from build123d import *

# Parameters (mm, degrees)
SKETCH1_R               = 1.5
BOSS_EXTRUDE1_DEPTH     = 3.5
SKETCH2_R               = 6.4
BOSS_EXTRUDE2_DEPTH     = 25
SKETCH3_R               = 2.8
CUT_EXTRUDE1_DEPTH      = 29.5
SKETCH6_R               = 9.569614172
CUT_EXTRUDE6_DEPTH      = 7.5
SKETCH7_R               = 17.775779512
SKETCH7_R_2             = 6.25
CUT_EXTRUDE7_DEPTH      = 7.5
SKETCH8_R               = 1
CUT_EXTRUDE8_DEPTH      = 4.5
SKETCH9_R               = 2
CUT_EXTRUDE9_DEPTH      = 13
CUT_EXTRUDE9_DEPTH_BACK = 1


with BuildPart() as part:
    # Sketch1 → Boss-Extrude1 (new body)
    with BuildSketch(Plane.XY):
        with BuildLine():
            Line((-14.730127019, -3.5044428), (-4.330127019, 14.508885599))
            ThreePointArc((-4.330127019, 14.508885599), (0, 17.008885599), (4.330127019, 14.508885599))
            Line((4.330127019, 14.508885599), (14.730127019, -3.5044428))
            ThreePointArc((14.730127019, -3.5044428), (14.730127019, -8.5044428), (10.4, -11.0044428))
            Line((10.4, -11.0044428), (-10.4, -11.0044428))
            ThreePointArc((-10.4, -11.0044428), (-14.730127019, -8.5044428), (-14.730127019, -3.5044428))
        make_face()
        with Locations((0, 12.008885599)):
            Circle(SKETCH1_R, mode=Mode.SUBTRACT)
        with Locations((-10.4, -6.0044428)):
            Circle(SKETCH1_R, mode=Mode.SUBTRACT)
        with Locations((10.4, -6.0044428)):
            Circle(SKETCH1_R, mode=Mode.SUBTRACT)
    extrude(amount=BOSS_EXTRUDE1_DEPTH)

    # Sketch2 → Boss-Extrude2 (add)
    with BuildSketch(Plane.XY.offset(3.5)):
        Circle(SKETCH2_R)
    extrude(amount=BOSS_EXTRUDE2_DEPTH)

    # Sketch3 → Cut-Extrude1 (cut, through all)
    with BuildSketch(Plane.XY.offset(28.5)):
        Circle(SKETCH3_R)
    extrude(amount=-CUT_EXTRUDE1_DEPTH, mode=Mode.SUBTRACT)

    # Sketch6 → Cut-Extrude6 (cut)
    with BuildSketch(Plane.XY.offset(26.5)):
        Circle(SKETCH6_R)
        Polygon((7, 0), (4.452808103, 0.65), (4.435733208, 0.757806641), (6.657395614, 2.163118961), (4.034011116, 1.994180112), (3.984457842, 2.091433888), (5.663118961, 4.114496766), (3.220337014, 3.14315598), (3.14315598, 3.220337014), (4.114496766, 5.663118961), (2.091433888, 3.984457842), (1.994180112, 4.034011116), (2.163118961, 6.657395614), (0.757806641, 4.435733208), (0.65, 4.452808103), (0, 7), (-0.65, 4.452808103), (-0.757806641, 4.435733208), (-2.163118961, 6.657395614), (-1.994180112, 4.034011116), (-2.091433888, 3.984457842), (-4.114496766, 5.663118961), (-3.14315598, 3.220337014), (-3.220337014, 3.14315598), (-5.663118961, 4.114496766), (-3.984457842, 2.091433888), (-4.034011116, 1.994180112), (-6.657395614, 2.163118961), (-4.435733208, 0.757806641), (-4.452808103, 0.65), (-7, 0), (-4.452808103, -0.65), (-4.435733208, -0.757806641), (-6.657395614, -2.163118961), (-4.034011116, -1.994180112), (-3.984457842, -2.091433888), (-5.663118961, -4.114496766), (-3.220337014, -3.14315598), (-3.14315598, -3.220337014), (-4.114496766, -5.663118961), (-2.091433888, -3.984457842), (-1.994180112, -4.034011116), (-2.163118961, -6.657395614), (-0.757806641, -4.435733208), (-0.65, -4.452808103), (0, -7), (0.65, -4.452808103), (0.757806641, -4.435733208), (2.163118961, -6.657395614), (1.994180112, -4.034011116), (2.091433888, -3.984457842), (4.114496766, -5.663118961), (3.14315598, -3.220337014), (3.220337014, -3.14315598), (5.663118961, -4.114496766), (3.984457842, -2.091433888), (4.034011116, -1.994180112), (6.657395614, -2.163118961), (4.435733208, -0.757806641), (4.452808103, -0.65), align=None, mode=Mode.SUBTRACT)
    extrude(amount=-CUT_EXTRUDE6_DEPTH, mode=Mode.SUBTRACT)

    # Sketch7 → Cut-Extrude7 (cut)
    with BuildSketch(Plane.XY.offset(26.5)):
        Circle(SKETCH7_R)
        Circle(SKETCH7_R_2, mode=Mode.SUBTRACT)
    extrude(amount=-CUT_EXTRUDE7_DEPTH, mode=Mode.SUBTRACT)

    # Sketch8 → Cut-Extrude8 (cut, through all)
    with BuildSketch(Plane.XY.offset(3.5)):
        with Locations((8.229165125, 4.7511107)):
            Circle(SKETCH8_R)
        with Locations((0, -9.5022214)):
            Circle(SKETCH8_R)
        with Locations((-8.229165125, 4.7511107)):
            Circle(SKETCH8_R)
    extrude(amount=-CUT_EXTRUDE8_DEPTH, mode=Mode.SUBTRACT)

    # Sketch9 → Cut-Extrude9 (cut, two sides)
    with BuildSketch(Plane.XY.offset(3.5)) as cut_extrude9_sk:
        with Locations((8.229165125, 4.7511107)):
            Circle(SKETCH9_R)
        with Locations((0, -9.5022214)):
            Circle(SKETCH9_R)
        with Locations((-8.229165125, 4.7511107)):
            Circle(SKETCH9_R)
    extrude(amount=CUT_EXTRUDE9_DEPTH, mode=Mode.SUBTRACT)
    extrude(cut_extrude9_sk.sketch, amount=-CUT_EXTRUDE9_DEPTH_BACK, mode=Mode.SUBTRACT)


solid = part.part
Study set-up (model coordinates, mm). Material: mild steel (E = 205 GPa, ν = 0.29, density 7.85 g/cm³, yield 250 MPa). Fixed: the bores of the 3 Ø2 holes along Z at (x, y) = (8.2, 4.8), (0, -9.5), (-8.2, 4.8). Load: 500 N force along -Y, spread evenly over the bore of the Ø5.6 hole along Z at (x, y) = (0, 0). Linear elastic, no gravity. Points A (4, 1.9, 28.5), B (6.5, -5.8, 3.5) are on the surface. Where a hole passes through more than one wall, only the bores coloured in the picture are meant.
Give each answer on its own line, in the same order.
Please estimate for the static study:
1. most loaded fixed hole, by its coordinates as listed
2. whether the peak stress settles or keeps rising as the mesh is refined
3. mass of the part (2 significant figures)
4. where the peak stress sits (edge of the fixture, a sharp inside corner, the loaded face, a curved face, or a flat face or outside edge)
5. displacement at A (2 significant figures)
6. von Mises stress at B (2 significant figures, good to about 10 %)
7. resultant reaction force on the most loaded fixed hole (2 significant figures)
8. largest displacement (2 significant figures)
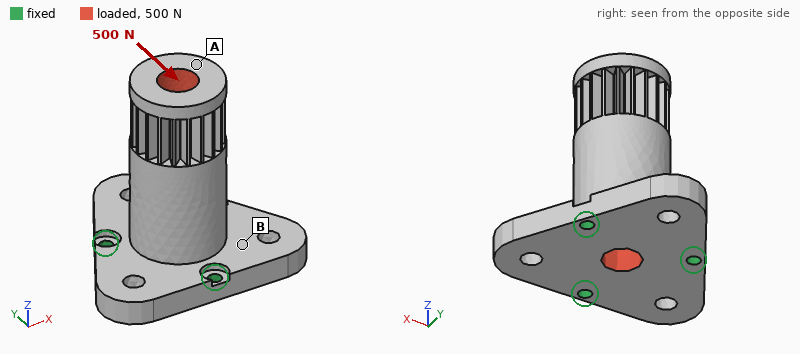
(0, -9.5)
keeps rising
32 g
edge of the fixture
12 µm
14 MPa
540 N
12 µm
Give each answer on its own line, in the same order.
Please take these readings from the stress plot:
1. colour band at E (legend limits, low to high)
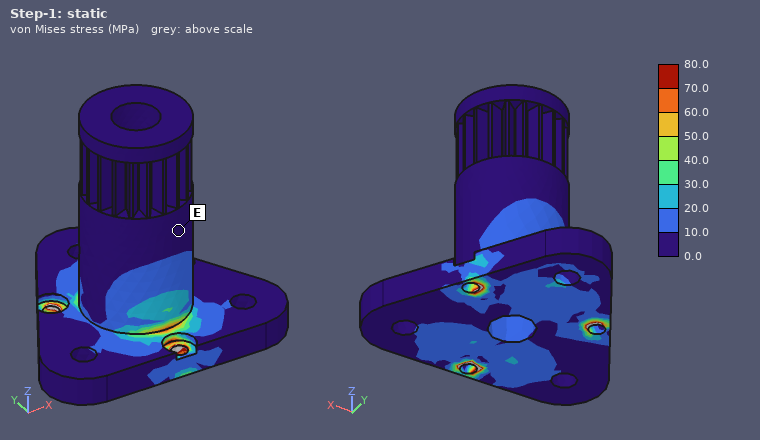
0.0 to 10.0 MPa
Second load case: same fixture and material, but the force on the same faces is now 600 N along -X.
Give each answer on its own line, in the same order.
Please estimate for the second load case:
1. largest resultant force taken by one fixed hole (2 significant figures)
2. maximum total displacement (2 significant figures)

560 N
15 µm
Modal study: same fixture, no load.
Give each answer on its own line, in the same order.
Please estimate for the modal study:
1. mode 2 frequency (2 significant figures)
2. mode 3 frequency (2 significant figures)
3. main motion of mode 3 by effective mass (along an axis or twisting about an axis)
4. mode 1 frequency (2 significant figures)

8800 Hz
21 kHz
along Z
8800 Hz
